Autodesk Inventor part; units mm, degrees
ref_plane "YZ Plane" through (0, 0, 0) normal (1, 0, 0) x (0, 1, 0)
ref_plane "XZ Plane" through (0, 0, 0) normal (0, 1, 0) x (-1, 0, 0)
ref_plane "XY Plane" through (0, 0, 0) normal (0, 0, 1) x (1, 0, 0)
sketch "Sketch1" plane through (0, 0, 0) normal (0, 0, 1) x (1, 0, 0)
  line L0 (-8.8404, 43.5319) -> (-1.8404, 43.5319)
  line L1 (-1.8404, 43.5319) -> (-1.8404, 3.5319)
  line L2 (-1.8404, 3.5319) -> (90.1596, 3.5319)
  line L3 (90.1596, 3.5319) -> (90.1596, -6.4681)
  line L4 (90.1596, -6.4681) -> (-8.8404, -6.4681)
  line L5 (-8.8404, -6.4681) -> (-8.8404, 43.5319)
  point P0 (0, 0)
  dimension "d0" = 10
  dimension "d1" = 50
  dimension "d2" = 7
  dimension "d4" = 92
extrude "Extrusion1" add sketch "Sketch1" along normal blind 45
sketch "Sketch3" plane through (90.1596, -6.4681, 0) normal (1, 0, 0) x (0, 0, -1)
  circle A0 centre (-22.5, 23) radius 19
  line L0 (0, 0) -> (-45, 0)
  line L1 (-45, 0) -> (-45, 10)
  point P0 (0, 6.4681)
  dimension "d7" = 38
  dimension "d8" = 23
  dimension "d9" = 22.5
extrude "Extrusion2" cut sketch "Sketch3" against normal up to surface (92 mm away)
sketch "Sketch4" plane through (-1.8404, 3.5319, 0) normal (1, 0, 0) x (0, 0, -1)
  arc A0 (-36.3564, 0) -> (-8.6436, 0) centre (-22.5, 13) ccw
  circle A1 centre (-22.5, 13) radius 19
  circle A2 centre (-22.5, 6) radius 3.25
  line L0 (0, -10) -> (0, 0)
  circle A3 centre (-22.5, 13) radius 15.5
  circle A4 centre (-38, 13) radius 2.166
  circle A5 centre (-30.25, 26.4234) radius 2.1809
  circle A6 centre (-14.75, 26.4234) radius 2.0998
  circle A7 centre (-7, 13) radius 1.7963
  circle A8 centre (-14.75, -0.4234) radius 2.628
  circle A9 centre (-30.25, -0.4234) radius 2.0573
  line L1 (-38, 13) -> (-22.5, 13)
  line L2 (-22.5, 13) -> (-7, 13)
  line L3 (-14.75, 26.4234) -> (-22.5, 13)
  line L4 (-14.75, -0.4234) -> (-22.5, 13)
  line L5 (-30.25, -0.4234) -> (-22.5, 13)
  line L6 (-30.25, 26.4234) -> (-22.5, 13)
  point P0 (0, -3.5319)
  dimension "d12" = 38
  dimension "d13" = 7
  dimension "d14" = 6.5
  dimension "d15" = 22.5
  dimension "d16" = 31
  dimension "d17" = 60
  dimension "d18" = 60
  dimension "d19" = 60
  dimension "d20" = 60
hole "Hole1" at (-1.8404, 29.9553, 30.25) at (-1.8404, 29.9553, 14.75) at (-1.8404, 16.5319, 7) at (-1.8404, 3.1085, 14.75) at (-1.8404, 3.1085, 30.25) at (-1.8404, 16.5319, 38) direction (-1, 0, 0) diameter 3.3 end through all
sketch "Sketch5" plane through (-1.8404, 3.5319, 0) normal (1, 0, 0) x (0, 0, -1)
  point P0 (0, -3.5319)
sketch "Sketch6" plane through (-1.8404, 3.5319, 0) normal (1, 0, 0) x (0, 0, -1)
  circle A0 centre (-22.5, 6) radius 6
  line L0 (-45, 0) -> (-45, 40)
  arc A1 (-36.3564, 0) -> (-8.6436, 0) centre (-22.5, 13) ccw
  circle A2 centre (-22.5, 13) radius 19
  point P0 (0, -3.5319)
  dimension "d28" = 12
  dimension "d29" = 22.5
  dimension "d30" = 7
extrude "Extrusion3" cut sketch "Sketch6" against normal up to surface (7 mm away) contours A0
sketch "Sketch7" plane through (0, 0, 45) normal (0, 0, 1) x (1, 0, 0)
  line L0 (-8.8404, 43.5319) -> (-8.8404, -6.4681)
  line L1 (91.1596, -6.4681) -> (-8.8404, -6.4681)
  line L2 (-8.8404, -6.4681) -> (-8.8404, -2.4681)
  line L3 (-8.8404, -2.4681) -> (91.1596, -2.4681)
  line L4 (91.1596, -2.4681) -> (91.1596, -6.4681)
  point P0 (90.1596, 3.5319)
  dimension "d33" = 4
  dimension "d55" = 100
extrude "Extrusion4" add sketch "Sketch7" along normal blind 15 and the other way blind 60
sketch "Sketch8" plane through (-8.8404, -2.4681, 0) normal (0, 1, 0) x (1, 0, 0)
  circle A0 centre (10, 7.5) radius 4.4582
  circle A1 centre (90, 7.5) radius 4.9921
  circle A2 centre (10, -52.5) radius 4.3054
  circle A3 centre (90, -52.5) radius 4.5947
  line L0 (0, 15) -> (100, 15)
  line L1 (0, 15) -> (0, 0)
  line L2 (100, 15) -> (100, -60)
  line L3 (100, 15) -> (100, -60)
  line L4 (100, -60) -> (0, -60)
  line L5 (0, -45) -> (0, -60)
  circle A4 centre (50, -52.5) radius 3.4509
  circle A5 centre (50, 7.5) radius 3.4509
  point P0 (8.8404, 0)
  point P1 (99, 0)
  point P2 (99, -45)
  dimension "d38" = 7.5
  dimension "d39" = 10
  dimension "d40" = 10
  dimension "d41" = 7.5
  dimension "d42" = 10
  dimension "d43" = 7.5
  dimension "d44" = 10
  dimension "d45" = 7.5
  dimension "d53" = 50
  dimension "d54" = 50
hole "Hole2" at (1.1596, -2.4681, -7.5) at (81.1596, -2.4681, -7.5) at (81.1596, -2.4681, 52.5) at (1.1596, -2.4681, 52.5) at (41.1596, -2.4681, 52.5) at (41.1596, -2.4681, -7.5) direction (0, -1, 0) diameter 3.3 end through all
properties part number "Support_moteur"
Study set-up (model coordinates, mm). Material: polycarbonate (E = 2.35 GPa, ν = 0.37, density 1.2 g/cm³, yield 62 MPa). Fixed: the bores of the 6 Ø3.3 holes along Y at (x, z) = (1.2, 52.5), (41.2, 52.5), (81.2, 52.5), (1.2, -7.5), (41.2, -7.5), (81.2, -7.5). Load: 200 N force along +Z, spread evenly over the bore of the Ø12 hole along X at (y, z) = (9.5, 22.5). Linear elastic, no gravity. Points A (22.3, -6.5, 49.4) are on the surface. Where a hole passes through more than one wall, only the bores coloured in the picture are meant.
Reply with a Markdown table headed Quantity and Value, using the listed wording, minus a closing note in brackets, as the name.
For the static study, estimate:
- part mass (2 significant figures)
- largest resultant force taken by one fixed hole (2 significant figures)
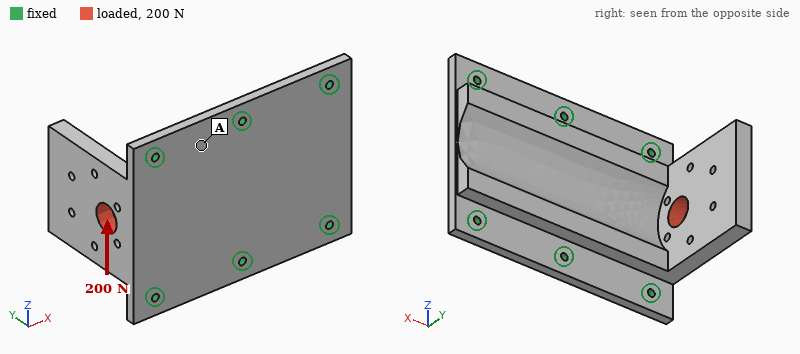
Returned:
| Quantity | Value |
|---|---|
| part mass | 69 g |
| largest resultant force taken by one fixed hole | 100 N |
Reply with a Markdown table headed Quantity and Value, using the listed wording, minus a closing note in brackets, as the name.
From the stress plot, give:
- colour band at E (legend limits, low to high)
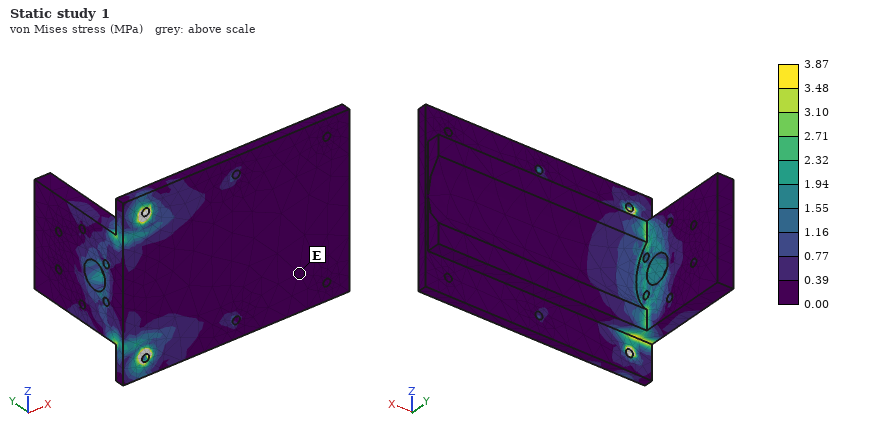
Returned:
| Quantity | Value |
|---|---|
| colour band at E | 0.00 to 0.39 MPa |
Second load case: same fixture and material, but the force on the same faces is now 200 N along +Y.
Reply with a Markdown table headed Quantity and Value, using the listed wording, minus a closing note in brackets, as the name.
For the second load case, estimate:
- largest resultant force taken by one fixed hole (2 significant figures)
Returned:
| Quantity | Value |
|---|---|
| largest resultant force taken by one fixed hole | 130 N |
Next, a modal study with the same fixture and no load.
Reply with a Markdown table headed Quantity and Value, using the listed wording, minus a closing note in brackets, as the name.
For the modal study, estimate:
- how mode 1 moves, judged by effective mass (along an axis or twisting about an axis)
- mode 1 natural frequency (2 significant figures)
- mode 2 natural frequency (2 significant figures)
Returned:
| Quantity | Value |
|---|---|
| how mode 1 moves, judged by effective mass | along X |
| mode 1 natural frequency | 550 Hz |
| mode 2 natural frequency | 1400 Hz |
